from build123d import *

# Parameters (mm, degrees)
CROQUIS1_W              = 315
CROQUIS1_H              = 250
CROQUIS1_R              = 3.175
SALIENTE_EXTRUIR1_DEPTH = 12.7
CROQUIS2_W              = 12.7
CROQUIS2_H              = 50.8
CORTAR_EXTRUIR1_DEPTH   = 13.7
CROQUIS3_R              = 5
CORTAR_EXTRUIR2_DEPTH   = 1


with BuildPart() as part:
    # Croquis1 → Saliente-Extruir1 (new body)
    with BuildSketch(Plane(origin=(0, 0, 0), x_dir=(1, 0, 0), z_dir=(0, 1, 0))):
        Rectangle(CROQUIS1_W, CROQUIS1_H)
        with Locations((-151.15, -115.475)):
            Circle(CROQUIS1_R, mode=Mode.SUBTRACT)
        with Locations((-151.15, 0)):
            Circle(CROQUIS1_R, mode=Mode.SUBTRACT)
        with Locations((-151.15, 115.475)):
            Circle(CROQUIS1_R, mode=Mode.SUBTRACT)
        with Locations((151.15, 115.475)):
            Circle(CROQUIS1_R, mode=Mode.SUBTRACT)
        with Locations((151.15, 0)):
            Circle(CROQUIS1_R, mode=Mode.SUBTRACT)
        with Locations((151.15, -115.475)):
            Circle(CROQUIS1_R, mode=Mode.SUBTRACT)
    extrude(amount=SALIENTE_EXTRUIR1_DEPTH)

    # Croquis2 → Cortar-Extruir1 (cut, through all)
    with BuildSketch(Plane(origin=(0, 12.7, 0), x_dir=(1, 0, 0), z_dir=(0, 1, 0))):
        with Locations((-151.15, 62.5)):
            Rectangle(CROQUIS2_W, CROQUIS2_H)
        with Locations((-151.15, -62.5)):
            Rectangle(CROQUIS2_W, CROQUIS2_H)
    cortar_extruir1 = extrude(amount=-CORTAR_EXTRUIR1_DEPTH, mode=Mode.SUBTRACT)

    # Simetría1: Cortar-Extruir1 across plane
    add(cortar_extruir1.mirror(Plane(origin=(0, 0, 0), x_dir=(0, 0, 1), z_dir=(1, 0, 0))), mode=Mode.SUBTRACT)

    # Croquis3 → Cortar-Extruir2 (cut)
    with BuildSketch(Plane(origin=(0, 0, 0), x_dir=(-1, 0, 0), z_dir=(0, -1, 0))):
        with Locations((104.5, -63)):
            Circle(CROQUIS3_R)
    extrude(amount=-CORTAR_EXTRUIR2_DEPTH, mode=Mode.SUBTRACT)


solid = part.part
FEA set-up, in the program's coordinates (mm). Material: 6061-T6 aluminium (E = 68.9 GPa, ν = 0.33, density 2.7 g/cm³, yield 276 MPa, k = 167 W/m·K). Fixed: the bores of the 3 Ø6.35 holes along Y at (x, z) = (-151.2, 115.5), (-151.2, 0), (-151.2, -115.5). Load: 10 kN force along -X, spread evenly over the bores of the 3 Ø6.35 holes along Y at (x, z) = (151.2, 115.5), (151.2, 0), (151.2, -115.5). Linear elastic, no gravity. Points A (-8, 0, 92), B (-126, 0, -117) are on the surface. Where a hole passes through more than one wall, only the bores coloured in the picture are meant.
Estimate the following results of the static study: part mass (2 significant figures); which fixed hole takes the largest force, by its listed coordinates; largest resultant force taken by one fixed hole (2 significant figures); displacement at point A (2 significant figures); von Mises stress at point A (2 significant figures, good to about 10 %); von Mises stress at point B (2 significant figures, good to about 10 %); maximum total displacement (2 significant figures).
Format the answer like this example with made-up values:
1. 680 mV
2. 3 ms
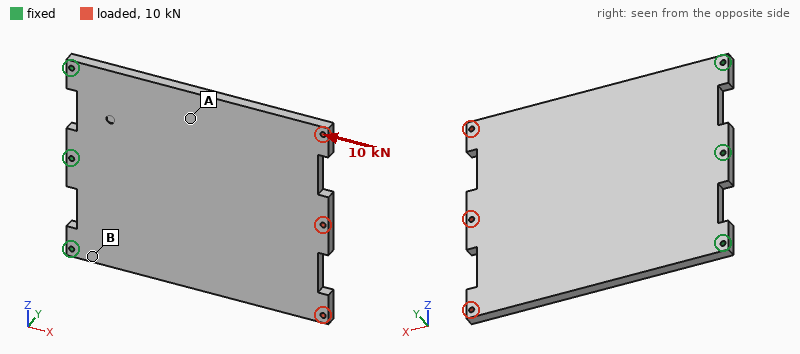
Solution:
1. 2.6 kg
2. (-151.2, 0)
3. 4.1 kN
4. 11 µm
5. 3.4 MPa
6. 7.3 MPa
7. 31 µm
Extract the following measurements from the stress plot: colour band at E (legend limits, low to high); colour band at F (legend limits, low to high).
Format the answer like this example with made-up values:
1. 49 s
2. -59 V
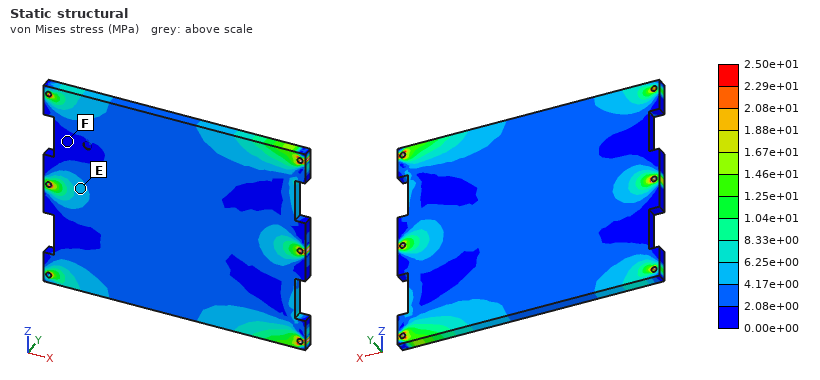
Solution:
1. 4.17e+00 to 6.25e+00 MPa
2. 0.00e+00 to 2.08e+00 MPa
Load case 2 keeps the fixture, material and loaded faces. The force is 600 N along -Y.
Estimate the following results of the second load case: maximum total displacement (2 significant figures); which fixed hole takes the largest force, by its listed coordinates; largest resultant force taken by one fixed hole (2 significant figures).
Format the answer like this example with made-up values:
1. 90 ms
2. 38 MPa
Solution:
1. 2.6 mm
2. (-151.2, 0)
3. 580 N
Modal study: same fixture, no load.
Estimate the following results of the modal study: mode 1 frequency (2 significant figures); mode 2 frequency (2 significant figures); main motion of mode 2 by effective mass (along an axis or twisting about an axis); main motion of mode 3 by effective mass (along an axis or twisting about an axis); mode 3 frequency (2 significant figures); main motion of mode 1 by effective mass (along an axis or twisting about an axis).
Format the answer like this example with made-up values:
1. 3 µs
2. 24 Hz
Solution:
1. 93 Hz
2. 300 Hz
3. twisting about X
4. along Y
5. 630 Hz
6. along Y
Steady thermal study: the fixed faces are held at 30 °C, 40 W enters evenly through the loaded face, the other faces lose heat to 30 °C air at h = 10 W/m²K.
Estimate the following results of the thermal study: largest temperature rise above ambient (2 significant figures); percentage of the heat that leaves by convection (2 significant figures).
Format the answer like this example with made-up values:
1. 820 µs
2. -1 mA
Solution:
1. 24 K
2. 40 %
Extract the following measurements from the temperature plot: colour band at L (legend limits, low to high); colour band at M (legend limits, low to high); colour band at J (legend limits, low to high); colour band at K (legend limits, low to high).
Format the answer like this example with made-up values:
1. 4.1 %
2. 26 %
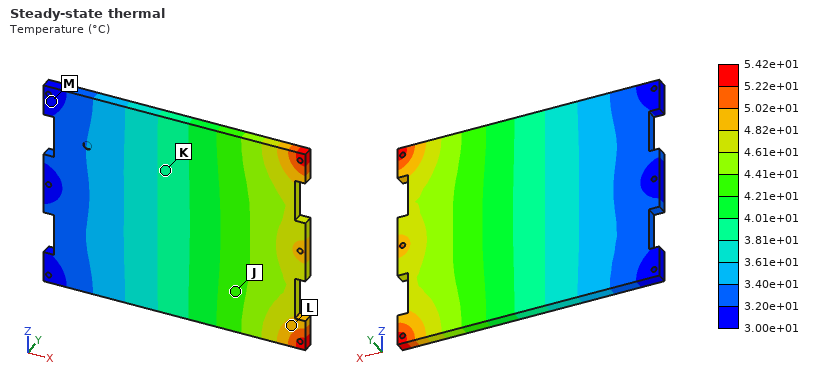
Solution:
1. 4.82e+01 to 5.02e+01 °C
2. 3.00e+01 to 3.20e+01 °C
3. 4.21e+01 to 4.41e+01 °C
4. 3.81e+01 to 4.01e+01 °C
